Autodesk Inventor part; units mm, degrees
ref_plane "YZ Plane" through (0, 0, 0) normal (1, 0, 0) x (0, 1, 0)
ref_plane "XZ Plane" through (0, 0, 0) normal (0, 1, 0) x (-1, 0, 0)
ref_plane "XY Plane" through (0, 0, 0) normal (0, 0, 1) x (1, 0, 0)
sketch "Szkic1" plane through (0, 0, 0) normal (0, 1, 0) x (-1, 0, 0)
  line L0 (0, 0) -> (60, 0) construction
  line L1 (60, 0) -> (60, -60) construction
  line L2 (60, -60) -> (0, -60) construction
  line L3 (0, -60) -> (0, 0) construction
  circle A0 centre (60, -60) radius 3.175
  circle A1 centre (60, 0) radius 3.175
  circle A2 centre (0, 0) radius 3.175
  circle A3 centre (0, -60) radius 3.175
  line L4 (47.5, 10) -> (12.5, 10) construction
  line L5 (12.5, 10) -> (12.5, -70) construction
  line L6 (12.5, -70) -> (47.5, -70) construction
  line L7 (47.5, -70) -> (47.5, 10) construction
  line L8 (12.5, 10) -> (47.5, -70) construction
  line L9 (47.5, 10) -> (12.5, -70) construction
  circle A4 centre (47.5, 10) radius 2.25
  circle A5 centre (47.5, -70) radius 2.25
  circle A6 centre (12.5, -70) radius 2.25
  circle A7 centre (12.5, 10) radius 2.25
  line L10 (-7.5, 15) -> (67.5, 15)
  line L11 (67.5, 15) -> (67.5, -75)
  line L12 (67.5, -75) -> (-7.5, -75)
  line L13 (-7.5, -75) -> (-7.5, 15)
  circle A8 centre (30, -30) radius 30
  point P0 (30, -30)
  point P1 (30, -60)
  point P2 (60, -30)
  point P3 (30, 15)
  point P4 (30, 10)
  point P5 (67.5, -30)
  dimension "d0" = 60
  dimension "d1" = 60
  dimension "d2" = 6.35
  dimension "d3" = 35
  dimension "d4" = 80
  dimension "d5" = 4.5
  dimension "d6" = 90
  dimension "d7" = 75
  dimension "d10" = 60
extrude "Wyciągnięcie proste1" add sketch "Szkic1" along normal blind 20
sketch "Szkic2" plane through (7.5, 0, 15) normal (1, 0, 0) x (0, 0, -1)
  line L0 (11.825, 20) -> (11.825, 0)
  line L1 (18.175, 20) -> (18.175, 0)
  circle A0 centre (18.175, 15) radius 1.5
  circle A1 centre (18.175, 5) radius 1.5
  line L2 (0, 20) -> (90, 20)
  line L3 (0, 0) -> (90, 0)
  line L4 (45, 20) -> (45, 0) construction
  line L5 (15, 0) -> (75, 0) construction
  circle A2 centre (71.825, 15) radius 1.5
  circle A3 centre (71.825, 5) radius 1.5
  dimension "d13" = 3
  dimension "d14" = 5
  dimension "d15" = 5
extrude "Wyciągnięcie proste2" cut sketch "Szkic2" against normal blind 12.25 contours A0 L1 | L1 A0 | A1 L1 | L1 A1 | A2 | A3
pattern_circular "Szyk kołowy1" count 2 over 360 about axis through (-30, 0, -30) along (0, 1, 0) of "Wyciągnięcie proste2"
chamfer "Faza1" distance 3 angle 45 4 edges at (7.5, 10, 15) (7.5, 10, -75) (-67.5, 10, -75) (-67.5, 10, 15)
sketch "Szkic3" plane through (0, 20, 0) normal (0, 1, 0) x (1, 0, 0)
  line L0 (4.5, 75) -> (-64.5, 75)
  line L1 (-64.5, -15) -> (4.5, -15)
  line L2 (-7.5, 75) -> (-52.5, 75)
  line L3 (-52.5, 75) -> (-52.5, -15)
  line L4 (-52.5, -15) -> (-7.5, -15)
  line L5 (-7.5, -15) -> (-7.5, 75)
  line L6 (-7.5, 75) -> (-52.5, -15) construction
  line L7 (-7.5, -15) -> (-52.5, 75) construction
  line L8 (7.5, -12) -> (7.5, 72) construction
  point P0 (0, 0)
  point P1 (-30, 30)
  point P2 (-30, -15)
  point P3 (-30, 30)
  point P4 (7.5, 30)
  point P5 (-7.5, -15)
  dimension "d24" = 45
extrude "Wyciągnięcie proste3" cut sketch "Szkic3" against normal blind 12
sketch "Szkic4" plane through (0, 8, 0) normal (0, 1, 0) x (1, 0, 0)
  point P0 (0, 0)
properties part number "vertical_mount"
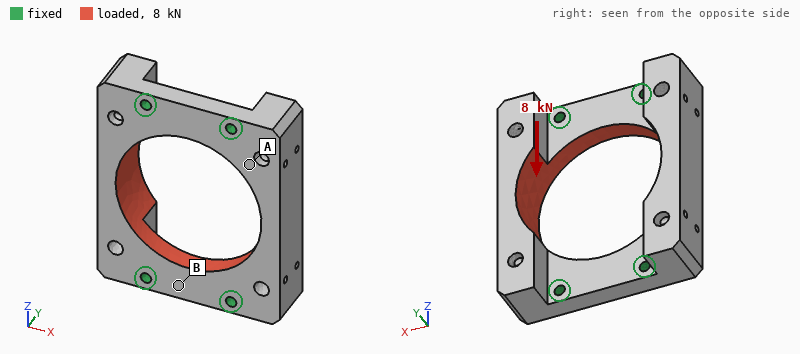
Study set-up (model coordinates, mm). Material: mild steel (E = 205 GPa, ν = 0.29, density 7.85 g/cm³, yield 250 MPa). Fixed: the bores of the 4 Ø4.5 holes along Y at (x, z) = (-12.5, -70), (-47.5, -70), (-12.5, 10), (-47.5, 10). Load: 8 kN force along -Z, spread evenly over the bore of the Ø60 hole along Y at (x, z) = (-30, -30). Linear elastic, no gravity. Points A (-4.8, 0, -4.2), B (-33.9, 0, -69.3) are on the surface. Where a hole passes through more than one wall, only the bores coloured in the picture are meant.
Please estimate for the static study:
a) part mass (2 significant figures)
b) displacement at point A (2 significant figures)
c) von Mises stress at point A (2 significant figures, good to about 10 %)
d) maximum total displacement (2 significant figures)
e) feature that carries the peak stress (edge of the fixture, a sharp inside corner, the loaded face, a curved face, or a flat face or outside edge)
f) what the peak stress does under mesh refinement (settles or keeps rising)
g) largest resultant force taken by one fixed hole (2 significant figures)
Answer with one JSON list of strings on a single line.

["430 g", "2.1 µm", "17 MPa", "4.0 µm", "edge of the fixture", "keeps rising", "2.0 kN"]
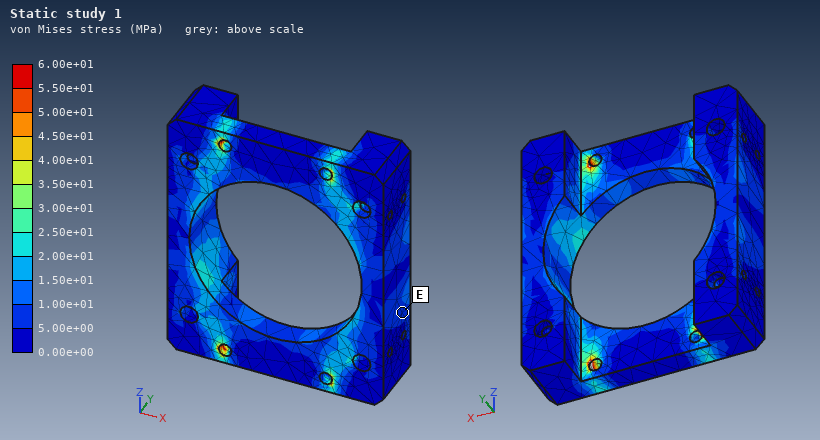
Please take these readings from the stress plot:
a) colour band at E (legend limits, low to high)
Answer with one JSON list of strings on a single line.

["5.00e+00 to 1.00e+01 MPa"]
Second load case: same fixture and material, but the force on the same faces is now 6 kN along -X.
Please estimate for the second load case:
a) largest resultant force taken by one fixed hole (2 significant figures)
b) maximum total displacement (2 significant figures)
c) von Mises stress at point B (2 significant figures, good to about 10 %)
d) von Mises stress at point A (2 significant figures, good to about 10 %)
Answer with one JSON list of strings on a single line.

["1.6 kN", "16 µm", "11 MPa", "9.2 MPa"]
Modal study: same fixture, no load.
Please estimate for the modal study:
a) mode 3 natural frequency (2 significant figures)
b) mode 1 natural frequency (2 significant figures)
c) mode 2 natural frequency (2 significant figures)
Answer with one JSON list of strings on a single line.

["9400 Hz", "4700 Hz", "4700 Hz"]
